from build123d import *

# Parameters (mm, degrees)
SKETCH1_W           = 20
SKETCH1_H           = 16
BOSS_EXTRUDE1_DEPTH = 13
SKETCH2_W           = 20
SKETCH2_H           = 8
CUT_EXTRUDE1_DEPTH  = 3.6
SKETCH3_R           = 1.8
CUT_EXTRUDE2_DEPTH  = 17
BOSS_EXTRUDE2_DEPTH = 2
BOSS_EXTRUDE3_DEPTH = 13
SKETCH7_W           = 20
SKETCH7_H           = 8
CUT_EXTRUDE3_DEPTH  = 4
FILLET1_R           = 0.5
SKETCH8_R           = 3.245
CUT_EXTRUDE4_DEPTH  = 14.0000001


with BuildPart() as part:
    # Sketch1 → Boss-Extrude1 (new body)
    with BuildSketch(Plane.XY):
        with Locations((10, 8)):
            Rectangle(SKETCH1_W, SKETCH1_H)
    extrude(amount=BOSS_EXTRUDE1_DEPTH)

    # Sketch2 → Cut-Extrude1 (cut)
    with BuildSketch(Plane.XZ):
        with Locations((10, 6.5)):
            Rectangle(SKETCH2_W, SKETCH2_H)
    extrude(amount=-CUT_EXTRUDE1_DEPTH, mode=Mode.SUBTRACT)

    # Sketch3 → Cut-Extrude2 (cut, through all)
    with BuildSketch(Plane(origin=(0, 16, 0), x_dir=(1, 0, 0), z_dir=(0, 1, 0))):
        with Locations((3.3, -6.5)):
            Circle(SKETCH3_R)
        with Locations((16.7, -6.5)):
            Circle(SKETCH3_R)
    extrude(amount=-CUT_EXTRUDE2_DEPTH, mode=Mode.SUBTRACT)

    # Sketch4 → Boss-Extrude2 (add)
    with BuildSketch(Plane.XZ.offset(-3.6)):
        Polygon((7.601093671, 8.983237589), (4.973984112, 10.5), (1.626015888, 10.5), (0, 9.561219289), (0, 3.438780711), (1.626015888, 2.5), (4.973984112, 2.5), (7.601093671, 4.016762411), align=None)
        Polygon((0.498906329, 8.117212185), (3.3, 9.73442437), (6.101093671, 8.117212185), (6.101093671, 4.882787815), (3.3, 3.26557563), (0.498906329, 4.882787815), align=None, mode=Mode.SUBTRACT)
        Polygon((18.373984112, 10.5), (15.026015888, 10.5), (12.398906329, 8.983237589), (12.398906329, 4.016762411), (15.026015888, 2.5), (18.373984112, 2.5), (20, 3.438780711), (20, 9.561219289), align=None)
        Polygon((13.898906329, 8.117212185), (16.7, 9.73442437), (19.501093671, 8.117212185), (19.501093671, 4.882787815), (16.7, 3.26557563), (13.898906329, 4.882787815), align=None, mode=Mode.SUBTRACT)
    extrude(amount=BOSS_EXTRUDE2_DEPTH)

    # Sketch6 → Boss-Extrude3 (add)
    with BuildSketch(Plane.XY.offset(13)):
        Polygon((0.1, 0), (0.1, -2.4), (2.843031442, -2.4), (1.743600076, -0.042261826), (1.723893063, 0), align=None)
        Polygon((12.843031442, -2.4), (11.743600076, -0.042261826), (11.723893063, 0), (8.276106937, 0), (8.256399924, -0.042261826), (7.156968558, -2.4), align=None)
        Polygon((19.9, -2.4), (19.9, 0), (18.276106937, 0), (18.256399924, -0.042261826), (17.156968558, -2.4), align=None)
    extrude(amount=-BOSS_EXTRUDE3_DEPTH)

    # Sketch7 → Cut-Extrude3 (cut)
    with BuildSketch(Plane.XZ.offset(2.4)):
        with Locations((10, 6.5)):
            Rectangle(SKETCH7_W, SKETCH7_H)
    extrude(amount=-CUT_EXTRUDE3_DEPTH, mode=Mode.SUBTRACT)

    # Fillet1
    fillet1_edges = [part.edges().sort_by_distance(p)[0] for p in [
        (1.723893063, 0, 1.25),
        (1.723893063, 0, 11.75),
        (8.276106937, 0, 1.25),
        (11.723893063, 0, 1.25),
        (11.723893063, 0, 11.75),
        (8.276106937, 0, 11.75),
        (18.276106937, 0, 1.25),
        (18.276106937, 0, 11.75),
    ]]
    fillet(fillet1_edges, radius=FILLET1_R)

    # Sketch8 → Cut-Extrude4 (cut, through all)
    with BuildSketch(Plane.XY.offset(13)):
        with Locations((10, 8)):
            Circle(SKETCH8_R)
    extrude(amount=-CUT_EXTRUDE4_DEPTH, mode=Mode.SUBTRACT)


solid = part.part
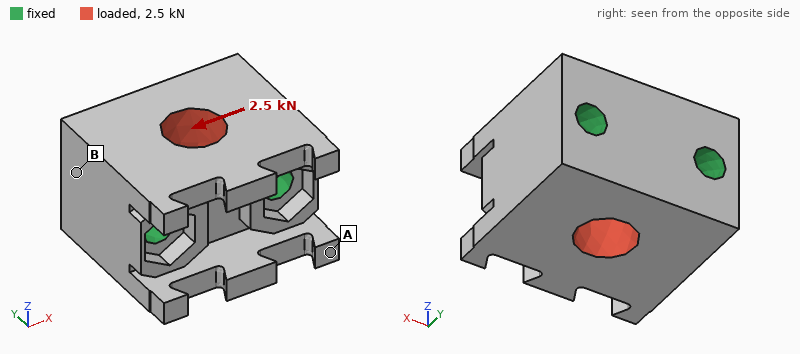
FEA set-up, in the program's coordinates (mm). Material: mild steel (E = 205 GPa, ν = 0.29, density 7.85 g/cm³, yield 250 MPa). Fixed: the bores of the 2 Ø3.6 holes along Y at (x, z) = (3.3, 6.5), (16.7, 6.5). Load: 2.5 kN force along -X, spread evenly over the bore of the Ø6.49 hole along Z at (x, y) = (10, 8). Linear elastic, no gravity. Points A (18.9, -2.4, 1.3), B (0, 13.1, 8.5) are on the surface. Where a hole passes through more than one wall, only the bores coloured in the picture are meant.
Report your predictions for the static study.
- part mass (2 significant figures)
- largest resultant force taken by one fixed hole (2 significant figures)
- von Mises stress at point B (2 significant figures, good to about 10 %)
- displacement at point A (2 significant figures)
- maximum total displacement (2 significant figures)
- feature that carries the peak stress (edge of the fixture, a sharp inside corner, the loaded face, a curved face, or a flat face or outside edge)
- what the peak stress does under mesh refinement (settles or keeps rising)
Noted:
25 g
1.3 kN
5.0 MPa
0.43 µm
0.53 µm
edge of the fixture
keeps rising
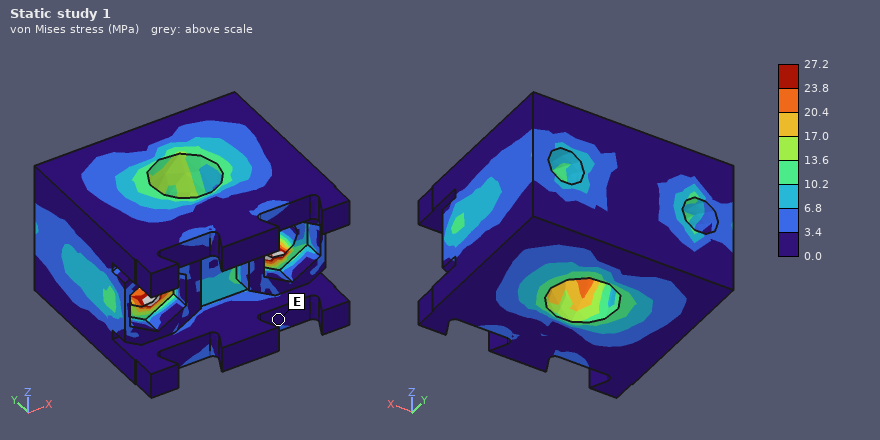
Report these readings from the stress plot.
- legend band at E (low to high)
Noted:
0.0 to 3.4 MPa
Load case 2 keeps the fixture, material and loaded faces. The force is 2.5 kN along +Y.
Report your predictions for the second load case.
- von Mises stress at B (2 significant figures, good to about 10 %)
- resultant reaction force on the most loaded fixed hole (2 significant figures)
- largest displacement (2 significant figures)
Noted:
3.0 MPa
1.3 kN
1.1 µm
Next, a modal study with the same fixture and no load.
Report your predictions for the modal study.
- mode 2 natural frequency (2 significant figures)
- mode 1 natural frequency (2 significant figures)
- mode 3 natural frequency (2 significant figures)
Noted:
47 kHz
45 kHz
60 kHz
